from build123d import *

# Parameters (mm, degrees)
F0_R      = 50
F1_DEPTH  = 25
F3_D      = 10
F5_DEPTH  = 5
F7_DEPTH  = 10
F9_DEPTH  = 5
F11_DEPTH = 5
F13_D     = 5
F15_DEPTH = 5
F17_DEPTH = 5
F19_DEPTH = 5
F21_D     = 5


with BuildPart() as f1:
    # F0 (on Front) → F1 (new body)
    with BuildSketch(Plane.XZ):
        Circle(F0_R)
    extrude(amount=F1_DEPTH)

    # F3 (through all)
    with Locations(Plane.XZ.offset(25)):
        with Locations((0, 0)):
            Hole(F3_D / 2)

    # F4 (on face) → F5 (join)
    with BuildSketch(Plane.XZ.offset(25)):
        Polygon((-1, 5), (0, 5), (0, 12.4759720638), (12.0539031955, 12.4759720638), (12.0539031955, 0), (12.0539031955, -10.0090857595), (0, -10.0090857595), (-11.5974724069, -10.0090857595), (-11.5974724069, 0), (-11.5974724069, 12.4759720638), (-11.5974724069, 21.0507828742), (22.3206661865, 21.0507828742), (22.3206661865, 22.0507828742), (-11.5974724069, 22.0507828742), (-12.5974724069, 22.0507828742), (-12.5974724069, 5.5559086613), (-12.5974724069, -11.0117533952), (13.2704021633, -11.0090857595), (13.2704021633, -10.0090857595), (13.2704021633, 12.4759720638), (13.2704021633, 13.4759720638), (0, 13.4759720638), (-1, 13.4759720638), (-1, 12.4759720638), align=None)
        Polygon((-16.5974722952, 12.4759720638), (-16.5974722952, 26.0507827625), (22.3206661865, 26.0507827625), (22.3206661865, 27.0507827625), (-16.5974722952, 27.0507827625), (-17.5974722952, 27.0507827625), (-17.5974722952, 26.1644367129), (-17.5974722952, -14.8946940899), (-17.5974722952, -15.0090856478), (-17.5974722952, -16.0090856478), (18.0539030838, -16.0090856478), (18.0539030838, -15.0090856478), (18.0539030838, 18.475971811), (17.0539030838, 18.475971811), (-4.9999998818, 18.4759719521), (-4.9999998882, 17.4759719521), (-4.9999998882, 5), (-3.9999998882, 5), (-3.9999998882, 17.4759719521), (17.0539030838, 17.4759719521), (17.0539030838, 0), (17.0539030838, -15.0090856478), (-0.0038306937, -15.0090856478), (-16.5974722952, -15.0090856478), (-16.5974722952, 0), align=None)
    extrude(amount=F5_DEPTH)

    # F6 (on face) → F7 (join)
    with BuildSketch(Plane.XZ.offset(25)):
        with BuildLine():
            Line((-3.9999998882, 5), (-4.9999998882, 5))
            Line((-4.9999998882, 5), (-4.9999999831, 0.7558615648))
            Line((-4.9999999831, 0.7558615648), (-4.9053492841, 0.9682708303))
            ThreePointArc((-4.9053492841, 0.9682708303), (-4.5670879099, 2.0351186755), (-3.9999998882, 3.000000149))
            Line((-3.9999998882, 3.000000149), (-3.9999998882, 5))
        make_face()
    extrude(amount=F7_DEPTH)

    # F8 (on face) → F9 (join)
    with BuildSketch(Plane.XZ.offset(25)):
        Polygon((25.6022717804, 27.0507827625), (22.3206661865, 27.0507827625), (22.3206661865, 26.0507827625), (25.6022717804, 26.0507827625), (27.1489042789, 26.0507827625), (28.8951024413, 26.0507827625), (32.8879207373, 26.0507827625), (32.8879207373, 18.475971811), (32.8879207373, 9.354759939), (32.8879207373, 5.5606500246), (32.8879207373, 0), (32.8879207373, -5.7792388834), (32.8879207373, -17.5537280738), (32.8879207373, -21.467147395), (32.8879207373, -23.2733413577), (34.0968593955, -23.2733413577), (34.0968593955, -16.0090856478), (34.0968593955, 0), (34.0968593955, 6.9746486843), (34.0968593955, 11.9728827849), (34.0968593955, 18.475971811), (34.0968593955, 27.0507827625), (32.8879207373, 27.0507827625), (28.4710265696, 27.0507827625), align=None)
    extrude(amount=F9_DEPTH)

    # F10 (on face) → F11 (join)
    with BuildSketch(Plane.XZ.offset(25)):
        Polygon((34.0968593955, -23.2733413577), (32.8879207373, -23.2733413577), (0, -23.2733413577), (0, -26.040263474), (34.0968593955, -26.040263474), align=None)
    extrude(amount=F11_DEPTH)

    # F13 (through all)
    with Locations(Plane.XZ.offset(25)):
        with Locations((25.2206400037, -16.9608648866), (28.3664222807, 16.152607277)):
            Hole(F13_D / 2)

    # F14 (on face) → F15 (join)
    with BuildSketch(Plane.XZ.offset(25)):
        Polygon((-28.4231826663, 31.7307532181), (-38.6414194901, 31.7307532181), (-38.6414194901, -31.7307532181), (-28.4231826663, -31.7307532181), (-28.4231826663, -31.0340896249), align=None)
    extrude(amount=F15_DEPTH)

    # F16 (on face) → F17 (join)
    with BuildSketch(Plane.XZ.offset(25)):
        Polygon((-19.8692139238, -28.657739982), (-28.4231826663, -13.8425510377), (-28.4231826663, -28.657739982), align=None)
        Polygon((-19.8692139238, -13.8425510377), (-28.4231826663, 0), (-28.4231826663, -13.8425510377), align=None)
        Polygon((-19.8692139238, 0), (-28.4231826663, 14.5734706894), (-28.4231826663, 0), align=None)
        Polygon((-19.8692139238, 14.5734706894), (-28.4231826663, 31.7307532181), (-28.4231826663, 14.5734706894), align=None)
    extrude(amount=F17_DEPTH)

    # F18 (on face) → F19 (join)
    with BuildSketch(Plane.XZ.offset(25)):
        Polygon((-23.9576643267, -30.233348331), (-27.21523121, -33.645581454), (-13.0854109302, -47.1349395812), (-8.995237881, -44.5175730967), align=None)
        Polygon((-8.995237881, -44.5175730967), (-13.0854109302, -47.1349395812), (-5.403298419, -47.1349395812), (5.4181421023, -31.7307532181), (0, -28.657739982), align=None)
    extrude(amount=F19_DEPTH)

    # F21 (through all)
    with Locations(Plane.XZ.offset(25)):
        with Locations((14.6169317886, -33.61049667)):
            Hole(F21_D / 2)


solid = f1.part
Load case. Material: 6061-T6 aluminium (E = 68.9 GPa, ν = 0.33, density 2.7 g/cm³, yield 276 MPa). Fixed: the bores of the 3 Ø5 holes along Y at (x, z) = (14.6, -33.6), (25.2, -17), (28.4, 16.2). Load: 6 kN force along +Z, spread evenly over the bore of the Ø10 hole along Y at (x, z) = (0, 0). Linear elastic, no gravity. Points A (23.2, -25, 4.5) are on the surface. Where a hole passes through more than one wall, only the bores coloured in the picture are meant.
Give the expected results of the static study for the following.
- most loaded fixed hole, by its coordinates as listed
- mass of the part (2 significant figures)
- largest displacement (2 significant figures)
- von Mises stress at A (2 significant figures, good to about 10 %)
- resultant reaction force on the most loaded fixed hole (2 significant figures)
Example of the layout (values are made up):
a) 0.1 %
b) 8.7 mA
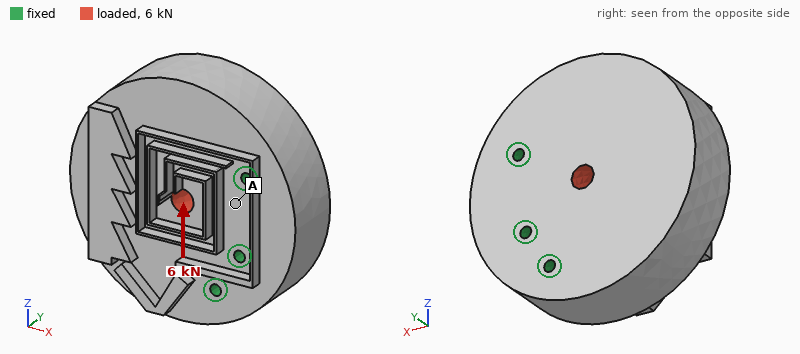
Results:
a) (14.6, -33.6)
b) 540 g
c) 6.1 µm
d) 3.9 MPa
e) 3.5 kN
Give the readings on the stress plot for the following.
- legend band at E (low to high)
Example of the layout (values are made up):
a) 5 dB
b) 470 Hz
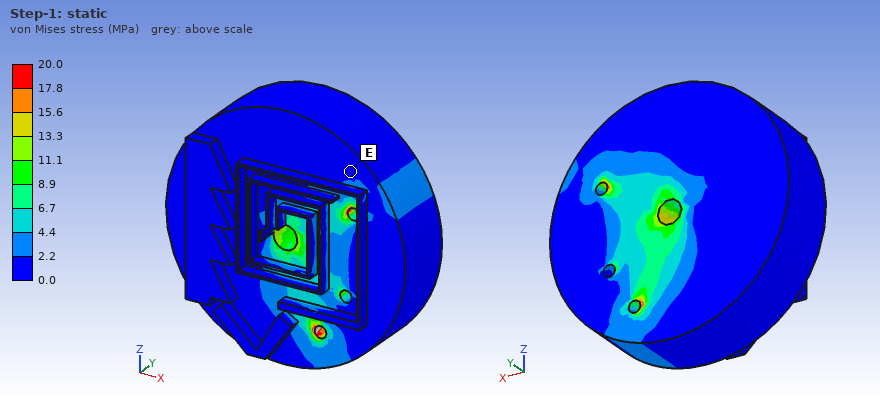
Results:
a) 0.0 to 2.2 MPa
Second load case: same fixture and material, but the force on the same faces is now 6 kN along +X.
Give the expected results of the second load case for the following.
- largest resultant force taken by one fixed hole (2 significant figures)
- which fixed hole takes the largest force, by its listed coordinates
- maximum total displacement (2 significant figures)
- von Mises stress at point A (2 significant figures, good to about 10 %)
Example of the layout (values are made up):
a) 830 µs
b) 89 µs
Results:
a) 3.4 kN
b) (28.4, 16.2)
c) 3.4 µm
d) 3.4 MPa
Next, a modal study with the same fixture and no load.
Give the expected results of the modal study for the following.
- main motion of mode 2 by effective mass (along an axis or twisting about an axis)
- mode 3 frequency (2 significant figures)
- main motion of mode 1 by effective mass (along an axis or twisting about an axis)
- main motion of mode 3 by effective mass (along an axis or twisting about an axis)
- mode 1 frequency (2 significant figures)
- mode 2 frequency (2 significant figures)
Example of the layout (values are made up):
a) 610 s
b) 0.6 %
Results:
a) along Z
b) 7200 Hz
c) along Y
d) twisting about X
e) 3500 Hz
f) 6600 Hz
